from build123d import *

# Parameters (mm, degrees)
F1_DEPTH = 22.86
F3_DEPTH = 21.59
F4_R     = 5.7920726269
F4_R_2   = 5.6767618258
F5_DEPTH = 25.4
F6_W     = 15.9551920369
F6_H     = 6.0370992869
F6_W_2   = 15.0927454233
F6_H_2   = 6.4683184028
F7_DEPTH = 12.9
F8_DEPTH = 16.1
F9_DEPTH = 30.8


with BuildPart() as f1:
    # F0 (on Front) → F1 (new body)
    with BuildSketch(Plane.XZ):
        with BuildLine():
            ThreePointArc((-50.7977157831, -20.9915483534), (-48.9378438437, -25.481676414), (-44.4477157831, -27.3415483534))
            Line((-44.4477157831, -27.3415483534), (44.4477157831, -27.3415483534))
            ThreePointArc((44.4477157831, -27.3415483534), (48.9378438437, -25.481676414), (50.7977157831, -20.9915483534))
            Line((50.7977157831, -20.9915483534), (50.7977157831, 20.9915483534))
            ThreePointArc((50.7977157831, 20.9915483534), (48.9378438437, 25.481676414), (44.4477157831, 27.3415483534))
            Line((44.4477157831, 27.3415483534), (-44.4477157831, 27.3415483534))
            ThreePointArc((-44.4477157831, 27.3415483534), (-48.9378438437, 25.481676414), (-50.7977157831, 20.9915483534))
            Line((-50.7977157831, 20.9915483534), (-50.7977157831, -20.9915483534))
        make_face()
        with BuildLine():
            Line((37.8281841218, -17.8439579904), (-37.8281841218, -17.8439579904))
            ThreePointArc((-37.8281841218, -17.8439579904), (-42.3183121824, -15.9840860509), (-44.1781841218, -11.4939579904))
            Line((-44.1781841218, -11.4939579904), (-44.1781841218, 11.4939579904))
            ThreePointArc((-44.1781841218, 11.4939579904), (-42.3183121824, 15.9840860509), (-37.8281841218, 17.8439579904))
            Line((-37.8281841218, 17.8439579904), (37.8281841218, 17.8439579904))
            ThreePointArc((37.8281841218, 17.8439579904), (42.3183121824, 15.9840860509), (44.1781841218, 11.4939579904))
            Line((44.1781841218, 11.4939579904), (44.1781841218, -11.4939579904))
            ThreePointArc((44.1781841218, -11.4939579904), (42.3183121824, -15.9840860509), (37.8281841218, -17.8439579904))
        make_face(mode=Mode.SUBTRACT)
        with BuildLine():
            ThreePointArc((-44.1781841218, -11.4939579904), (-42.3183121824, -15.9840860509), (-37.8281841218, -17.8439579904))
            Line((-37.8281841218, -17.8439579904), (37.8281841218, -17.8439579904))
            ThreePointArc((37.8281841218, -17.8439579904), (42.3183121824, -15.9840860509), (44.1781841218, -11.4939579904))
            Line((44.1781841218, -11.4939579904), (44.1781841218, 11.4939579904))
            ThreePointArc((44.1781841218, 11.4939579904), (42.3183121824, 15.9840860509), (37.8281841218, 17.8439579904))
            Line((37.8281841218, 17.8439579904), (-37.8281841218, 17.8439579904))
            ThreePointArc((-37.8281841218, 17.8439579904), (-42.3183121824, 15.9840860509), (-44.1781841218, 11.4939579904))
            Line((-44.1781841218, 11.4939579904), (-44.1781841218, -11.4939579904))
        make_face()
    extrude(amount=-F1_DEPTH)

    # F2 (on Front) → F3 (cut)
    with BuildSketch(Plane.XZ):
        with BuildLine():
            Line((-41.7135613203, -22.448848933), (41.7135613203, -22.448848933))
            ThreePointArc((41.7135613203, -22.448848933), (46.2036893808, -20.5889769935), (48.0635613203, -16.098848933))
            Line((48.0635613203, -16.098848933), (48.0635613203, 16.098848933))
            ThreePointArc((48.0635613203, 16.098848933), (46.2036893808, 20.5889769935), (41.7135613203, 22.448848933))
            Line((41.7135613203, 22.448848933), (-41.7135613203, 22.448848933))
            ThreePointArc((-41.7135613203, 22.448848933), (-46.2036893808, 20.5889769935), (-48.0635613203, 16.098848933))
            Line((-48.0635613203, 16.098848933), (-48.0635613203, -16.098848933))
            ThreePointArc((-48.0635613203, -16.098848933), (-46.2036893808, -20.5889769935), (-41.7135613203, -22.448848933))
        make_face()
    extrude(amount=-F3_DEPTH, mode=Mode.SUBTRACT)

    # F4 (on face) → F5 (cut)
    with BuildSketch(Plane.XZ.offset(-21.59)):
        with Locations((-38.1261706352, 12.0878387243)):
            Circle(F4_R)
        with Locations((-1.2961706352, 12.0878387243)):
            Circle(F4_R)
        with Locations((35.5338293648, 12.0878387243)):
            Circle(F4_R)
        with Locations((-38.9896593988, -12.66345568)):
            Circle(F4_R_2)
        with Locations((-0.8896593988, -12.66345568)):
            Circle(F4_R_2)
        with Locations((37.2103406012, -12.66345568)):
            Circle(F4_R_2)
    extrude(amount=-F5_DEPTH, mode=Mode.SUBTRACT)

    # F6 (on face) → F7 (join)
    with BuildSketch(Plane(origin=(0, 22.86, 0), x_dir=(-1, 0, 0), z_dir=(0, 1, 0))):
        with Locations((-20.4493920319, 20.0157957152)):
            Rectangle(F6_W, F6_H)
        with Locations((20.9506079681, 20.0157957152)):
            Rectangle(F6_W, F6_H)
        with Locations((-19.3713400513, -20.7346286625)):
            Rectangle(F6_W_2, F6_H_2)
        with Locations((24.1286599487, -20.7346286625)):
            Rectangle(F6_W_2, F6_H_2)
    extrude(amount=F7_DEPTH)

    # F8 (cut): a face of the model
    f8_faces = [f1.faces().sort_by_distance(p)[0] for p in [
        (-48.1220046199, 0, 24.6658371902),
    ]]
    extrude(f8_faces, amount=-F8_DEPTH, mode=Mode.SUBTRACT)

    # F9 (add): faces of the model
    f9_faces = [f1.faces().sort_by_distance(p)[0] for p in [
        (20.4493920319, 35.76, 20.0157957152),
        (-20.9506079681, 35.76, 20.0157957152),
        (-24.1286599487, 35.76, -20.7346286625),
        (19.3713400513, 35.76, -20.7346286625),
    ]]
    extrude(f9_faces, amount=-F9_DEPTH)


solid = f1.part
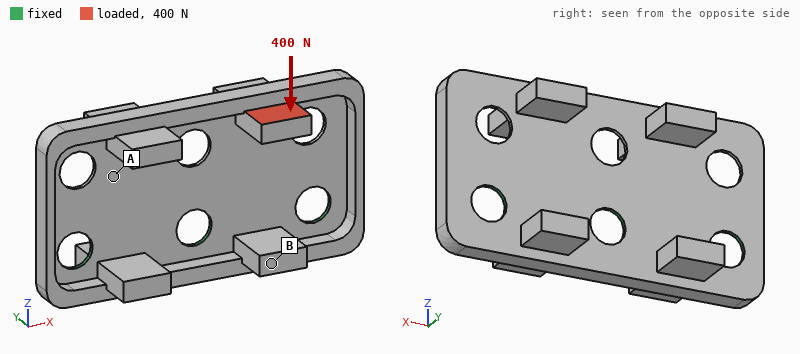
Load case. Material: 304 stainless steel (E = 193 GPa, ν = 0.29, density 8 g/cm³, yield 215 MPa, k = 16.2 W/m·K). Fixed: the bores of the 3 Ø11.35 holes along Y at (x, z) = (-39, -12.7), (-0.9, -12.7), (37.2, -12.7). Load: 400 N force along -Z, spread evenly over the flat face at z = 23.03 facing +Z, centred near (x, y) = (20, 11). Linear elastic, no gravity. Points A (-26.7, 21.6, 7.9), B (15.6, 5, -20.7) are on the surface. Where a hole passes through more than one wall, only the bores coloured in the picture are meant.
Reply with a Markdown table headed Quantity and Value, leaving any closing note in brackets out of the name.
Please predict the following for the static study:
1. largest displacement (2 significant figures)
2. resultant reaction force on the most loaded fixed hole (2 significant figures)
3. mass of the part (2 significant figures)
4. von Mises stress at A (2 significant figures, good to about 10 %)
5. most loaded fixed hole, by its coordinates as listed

| Quantity | Value |
|---|---|
| largest displacement | 0.21 mm |
| resultant reaction force on the most loaded fixed hole | 270 N |
| mass of the part | 190 g |
| von Mises stress at A | 22 MPa |
| most loaded fixed hole, by its coordinates as listed | (37.2, -12.7) |
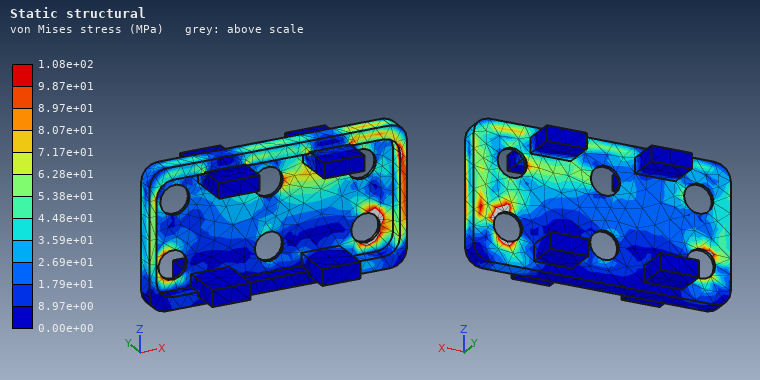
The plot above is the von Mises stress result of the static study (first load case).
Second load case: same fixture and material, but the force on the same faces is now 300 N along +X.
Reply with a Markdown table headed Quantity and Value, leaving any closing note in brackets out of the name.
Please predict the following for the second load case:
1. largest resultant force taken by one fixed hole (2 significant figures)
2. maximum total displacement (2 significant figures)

| Quantity | Value |
|---|---|
| largest resultant force taken by one fixed hole | 190 N |
| maximum total displacement | 49 µm |
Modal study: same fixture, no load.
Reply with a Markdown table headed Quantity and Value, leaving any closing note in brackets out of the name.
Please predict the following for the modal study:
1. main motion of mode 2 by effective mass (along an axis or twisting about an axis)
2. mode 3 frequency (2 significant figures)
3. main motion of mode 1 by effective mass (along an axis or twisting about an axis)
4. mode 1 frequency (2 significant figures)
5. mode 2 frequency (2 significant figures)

| Quantity | Value |
|---|---|
| main motion of mode 2 by effective mass | twisting about Z |
| mode 3 frequency | 2400 Hz |
| main motion of mode 1 by effective mass | along Y |
| mode 1 frequency | 660 Hz |
| mode 2 frequency | 1400 Hz |
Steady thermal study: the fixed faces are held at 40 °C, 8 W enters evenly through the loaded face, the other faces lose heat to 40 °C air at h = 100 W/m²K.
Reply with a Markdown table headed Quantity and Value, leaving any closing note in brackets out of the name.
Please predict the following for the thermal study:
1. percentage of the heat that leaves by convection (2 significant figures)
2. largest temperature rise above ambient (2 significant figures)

| Quantity | Value |
|---|---|
| percentage of the heat that leaves by convection | 98 % |
| largest temperature rise above ambient | 64 K |
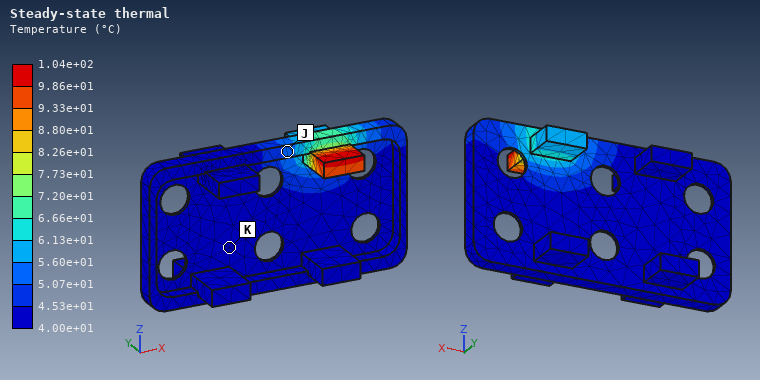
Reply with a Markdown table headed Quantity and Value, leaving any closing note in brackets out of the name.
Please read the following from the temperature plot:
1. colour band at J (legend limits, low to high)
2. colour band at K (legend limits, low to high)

| Quantity | Value |
|---|---|
| colour band at J | 5.07e+01 to 5.60e+01 °C |
| colour band at K | 4.00e+01 to 4.53e+01 °C |
